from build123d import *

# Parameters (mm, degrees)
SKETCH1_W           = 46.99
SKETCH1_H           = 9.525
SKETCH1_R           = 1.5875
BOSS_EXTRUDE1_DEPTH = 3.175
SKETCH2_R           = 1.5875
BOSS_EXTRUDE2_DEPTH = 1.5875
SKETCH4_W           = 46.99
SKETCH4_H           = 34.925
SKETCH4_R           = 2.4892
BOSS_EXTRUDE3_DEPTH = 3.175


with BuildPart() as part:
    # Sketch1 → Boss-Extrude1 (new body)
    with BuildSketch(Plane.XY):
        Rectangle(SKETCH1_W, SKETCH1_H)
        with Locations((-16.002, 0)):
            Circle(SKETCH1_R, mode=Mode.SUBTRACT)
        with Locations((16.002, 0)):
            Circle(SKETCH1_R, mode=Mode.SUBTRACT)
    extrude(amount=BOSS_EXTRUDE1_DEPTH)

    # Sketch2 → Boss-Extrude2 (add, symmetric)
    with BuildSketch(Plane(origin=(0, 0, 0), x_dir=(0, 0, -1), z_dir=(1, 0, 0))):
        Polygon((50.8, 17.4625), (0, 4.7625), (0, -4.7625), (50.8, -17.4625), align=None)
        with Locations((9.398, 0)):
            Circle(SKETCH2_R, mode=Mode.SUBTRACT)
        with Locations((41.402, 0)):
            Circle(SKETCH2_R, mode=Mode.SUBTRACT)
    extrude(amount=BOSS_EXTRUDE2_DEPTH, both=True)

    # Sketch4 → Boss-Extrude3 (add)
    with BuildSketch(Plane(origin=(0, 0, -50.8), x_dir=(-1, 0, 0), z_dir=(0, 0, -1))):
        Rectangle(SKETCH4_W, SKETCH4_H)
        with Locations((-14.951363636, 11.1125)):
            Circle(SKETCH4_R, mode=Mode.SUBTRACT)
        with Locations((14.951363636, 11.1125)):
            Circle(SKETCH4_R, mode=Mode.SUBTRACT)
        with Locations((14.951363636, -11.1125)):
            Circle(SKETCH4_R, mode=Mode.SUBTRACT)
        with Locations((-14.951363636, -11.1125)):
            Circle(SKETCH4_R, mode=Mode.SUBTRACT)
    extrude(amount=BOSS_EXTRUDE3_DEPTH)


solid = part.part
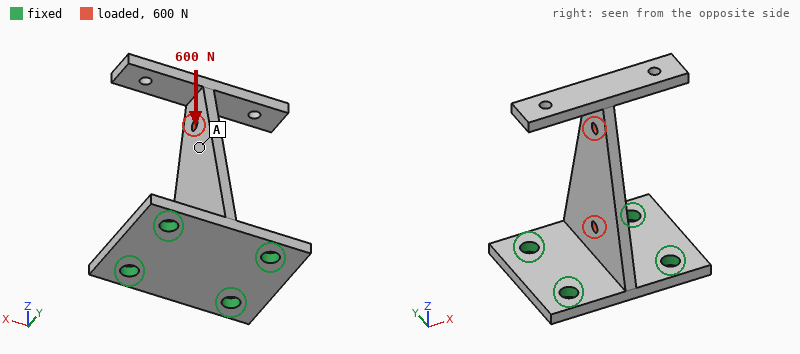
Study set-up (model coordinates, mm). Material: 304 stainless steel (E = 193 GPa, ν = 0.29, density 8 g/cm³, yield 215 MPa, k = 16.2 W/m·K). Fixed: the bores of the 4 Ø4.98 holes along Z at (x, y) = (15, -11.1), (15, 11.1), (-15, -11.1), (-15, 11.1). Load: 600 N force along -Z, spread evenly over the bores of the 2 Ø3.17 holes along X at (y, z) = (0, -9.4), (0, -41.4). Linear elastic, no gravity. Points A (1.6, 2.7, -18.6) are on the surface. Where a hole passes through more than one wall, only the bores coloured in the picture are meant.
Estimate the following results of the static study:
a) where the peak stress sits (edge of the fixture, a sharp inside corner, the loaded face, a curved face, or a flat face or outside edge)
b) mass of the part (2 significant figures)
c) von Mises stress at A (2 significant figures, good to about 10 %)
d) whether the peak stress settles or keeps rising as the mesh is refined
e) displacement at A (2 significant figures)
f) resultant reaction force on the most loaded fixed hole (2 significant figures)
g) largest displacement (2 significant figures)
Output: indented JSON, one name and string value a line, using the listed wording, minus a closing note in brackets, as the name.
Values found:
{
  "where the peak stress sits": "edge of the fixture",
  "mass of the part": "79 g",
  "von Mises stress at A": "5.6 MPa",
  "whether the peak stress settles or keeps rising as the mesh is refined": "keeps rising",
  "displacement at A": "4.8 µm",
  "resultant reaction force on the most loaded fixed hole": "150 N",
  "largest displacement": "5.2 µm"
}
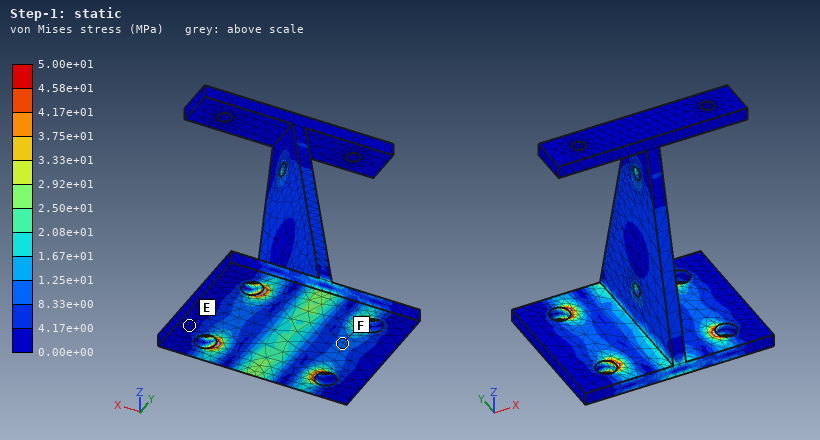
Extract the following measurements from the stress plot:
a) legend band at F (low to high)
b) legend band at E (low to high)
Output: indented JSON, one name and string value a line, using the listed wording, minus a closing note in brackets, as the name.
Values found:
{
  "legend band at F": "8.33e+00 to 1.25e+01 MPa",
  "legend band at E": "0.00e+00 to 4.17e+00 MPa"
}
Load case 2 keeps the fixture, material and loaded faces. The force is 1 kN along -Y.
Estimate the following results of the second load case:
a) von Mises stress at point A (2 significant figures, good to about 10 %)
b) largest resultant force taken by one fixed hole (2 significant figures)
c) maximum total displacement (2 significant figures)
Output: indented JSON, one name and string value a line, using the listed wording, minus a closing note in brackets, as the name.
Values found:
{
  "von Mises stress at point A": "17 MPa",
  "largest resultant force taken by one fixed hole": "630 N",
  "maximum total displacement": "93 µm"
}
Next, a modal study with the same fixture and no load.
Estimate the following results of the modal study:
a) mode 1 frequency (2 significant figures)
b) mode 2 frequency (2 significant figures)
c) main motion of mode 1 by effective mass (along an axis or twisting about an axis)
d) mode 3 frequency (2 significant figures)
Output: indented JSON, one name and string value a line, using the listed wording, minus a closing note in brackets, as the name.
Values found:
{
  "mode 1 frequency": "630 Hz",
  "mode 2 frequency": "1800 Hz",
  "main motion of mode 1 by effective mass": "along X",
  "mode 3 frequency": "2200 Hz"
}
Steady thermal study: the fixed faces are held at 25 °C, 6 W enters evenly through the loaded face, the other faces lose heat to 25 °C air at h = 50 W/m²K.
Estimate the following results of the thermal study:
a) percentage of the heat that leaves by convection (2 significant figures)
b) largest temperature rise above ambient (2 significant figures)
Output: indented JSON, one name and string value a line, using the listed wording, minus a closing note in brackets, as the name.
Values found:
{
  "percentage of the heat that leaves by convection": "72 %",
  "largest temperature rise above ambient": "47 K"
}
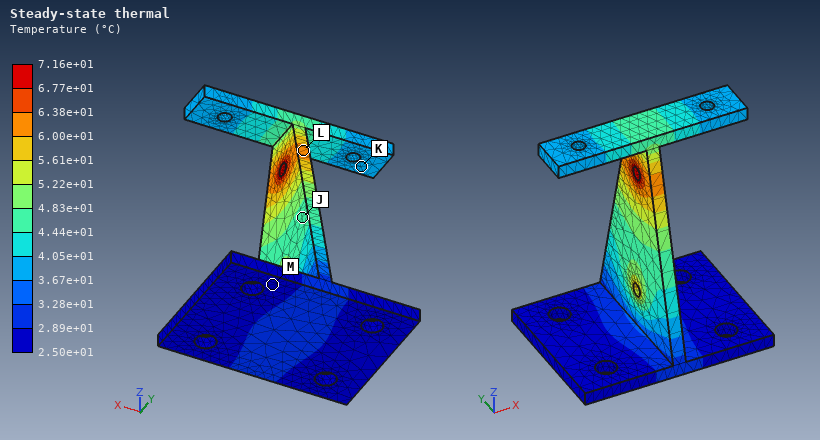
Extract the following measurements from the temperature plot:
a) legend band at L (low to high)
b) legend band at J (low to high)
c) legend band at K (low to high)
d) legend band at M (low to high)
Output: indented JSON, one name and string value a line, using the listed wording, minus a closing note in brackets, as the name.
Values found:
{
  "legend band at L": "6.00e+01 to 6.38e+01 °C",
  "legend band at J": "4.44e+01 to 4.83e+01 °C",
  "legend band at K": "3.67e+01 to 4.05e+01 °C",
  "legend band at M": "2.50e+01 to 2.89e+01 °C"
}
